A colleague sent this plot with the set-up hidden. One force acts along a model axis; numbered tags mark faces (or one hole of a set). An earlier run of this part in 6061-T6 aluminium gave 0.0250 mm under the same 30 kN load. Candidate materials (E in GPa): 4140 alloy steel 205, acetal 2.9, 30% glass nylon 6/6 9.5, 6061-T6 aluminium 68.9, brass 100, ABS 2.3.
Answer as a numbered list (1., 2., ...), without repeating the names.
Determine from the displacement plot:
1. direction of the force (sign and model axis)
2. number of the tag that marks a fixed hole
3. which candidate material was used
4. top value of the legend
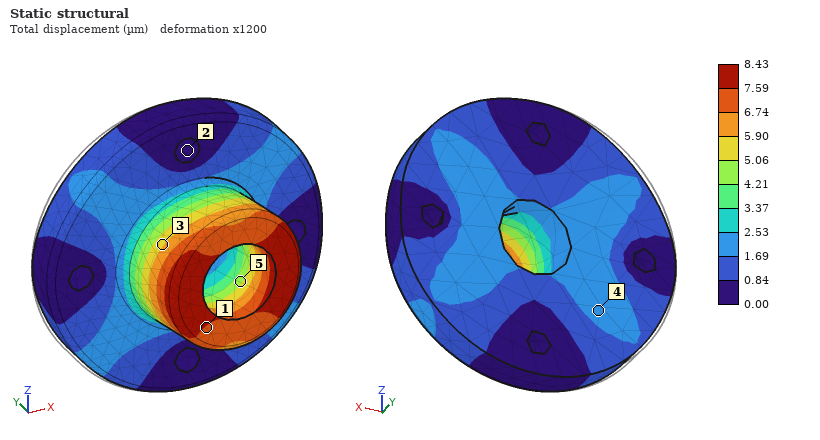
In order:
1. +X
2. 2
3. 4140 alloy steel
4. 8.43 µm
